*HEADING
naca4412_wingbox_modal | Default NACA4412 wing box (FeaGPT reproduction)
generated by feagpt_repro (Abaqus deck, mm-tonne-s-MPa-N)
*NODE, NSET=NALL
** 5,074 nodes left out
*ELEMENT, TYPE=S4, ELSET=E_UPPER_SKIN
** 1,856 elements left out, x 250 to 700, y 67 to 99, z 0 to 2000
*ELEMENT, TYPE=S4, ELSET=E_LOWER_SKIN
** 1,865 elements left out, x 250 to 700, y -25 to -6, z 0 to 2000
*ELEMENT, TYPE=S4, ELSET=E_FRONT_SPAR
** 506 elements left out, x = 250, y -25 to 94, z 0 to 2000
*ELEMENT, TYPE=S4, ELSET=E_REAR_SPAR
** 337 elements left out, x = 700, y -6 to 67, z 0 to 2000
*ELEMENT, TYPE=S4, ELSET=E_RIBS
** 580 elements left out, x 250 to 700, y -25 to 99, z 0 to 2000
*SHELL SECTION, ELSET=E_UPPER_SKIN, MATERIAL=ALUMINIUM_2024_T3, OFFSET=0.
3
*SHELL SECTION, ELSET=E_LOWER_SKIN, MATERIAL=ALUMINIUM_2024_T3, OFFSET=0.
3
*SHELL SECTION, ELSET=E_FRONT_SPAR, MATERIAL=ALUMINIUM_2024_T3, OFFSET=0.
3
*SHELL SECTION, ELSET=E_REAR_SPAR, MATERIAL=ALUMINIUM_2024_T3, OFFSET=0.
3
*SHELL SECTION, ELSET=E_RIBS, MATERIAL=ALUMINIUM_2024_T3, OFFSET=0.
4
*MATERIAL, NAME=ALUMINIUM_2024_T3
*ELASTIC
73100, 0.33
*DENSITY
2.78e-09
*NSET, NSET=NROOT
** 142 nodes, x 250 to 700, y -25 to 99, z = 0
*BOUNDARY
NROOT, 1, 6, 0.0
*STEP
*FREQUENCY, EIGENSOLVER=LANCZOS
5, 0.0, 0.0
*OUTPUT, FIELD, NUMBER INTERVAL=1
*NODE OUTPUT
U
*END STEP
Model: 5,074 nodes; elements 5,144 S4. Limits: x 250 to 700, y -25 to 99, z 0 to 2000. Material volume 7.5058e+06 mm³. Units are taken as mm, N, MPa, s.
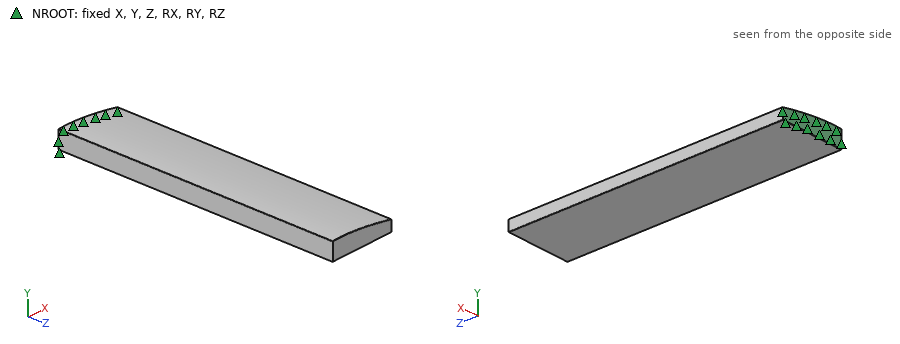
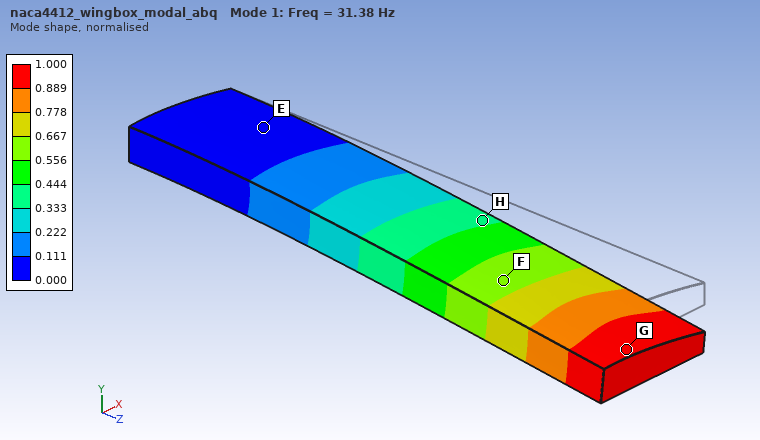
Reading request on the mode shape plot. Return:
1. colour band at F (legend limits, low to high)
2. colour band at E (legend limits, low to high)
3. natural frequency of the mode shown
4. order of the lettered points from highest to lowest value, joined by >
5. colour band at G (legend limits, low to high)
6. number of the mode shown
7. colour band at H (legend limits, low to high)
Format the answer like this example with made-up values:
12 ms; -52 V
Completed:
0.556 to 0.667; 0.000 to 0.111; 31.38 Hz; G > F > H > E; 0.889 to 1.000; 1; 0.333 to 0.444
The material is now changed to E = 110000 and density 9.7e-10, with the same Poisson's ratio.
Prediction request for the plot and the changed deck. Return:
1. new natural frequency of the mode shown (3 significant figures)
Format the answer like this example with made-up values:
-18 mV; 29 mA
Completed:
65.2 Hz
